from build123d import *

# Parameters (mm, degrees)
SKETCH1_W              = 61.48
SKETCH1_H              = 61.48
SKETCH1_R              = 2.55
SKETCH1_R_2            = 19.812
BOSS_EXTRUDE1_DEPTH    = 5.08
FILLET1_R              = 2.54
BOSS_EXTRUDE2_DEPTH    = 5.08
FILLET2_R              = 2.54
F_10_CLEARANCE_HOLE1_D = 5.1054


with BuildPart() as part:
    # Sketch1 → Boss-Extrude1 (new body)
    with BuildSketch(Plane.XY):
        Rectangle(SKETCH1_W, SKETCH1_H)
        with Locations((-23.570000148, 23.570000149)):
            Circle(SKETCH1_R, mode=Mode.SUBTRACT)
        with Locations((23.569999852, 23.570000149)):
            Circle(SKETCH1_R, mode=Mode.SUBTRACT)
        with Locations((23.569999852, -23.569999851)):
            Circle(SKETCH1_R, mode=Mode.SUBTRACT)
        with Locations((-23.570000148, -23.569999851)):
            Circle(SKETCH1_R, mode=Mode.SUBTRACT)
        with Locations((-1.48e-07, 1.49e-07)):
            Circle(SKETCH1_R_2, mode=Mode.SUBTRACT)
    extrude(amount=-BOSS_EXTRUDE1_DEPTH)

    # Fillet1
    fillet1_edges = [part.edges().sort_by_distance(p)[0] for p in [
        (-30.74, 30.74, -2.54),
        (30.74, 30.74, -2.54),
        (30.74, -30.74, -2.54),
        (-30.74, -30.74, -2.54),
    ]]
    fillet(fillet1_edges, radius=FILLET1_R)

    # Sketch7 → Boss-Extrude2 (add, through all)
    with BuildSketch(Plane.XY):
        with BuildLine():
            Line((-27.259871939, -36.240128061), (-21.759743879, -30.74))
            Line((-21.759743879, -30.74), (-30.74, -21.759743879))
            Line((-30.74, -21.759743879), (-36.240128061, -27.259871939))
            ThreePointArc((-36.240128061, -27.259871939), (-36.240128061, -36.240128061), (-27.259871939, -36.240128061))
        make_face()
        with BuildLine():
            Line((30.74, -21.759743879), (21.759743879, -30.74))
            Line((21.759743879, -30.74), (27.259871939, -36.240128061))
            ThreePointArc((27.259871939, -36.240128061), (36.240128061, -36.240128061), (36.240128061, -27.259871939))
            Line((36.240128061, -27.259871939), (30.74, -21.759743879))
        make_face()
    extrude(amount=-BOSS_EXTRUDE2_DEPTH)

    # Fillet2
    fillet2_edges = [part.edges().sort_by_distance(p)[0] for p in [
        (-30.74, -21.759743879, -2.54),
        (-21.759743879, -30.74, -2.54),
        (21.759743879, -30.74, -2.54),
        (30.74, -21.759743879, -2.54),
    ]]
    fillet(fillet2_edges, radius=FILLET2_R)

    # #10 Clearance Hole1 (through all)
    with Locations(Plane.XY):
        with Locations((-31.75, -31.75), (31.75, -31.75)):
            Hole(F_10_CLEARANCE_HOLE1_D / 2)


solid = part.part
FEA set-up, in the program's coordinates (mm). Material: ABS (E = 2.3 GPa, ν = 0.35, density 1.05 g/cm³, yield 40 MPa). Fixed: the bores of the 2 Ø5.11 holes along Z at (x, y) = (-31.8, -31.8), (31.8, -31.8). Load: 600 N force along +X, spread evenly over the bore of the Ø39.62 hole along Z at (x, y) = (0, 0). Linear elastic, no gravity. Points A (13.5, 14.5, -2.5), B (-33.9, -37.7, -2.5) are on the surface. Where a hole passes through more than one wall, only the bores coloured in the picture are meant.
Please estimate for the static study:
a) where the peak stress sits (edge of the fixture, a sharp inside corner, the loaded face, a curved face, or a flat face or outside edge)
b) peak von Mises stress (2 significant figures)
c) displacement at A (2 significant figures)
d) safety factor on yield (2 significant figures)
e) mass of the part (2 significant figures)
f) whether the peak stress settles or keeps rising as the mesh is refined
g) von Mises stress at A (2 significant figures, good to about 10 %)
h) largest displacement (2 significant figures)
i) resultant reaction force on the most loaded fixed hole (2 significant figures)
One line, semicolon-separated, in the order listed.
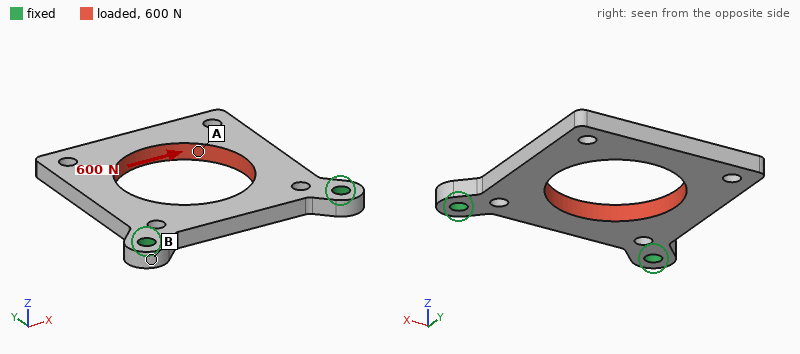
a curved face; 27 MPa; 0.60 mm; 1.5; 14 g; settles; 12 MPa; 0.66 mm; 410 N
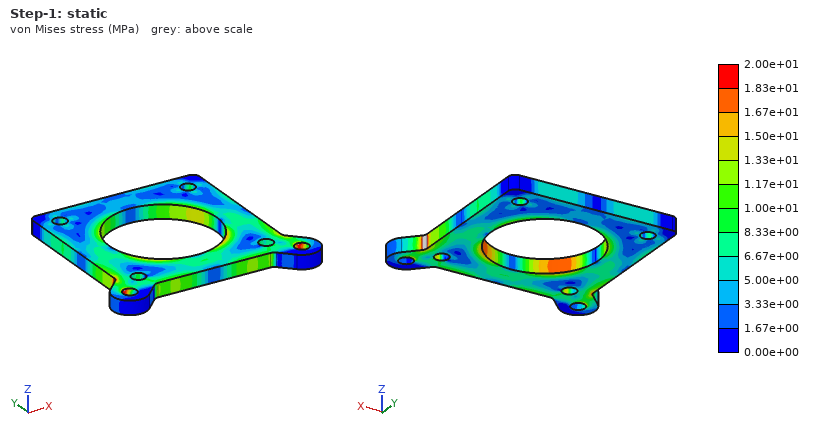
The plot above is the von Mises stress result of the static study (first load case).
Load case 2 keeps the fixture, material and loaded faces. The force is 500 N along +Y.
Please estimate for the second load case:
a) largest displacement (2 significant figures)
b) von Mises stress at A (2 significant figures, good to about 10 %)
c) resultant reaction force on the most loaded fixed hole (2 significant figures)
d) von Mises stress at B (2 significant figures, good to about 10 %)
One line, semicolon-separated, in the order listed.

0.11 mm; 3.0 MPa; 280 N; 1.3 MPa
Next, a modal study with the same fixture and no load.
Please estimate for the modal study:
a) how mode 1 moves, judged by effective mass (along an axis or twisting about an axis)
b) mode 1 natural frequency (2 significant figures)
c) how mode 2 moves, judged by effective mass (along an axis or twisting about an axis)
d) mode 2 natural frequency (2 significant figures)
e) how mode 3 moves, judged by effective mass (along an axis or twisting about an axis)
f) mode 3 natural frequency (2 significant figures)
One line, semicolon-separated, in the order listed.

along Z; 220 Hz; twisting about Y; 610 Hz; along X; 1400 Hz
